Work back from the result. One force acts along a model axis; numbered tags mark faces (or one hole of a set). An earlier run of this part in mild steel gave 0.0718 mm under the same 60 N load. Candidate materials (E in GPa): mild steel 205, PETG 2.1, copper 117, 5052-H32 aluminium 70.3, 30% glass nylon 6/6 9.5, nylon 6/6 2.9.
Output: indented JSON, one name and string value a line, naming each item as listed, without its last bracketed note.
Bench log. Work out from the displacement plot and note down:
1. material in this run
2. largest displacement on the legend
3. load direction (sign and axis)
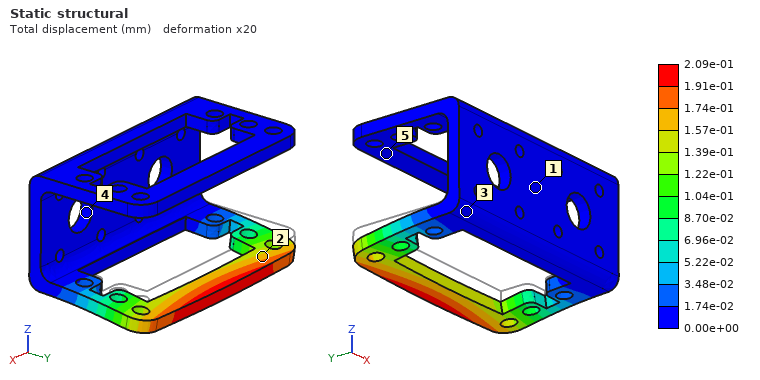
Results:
{
  "material in this run": "5052-H32 aluminium",
  "largest displacement on the legend": "2.09e-01 mm",
  "load direction": "-Z"
}
